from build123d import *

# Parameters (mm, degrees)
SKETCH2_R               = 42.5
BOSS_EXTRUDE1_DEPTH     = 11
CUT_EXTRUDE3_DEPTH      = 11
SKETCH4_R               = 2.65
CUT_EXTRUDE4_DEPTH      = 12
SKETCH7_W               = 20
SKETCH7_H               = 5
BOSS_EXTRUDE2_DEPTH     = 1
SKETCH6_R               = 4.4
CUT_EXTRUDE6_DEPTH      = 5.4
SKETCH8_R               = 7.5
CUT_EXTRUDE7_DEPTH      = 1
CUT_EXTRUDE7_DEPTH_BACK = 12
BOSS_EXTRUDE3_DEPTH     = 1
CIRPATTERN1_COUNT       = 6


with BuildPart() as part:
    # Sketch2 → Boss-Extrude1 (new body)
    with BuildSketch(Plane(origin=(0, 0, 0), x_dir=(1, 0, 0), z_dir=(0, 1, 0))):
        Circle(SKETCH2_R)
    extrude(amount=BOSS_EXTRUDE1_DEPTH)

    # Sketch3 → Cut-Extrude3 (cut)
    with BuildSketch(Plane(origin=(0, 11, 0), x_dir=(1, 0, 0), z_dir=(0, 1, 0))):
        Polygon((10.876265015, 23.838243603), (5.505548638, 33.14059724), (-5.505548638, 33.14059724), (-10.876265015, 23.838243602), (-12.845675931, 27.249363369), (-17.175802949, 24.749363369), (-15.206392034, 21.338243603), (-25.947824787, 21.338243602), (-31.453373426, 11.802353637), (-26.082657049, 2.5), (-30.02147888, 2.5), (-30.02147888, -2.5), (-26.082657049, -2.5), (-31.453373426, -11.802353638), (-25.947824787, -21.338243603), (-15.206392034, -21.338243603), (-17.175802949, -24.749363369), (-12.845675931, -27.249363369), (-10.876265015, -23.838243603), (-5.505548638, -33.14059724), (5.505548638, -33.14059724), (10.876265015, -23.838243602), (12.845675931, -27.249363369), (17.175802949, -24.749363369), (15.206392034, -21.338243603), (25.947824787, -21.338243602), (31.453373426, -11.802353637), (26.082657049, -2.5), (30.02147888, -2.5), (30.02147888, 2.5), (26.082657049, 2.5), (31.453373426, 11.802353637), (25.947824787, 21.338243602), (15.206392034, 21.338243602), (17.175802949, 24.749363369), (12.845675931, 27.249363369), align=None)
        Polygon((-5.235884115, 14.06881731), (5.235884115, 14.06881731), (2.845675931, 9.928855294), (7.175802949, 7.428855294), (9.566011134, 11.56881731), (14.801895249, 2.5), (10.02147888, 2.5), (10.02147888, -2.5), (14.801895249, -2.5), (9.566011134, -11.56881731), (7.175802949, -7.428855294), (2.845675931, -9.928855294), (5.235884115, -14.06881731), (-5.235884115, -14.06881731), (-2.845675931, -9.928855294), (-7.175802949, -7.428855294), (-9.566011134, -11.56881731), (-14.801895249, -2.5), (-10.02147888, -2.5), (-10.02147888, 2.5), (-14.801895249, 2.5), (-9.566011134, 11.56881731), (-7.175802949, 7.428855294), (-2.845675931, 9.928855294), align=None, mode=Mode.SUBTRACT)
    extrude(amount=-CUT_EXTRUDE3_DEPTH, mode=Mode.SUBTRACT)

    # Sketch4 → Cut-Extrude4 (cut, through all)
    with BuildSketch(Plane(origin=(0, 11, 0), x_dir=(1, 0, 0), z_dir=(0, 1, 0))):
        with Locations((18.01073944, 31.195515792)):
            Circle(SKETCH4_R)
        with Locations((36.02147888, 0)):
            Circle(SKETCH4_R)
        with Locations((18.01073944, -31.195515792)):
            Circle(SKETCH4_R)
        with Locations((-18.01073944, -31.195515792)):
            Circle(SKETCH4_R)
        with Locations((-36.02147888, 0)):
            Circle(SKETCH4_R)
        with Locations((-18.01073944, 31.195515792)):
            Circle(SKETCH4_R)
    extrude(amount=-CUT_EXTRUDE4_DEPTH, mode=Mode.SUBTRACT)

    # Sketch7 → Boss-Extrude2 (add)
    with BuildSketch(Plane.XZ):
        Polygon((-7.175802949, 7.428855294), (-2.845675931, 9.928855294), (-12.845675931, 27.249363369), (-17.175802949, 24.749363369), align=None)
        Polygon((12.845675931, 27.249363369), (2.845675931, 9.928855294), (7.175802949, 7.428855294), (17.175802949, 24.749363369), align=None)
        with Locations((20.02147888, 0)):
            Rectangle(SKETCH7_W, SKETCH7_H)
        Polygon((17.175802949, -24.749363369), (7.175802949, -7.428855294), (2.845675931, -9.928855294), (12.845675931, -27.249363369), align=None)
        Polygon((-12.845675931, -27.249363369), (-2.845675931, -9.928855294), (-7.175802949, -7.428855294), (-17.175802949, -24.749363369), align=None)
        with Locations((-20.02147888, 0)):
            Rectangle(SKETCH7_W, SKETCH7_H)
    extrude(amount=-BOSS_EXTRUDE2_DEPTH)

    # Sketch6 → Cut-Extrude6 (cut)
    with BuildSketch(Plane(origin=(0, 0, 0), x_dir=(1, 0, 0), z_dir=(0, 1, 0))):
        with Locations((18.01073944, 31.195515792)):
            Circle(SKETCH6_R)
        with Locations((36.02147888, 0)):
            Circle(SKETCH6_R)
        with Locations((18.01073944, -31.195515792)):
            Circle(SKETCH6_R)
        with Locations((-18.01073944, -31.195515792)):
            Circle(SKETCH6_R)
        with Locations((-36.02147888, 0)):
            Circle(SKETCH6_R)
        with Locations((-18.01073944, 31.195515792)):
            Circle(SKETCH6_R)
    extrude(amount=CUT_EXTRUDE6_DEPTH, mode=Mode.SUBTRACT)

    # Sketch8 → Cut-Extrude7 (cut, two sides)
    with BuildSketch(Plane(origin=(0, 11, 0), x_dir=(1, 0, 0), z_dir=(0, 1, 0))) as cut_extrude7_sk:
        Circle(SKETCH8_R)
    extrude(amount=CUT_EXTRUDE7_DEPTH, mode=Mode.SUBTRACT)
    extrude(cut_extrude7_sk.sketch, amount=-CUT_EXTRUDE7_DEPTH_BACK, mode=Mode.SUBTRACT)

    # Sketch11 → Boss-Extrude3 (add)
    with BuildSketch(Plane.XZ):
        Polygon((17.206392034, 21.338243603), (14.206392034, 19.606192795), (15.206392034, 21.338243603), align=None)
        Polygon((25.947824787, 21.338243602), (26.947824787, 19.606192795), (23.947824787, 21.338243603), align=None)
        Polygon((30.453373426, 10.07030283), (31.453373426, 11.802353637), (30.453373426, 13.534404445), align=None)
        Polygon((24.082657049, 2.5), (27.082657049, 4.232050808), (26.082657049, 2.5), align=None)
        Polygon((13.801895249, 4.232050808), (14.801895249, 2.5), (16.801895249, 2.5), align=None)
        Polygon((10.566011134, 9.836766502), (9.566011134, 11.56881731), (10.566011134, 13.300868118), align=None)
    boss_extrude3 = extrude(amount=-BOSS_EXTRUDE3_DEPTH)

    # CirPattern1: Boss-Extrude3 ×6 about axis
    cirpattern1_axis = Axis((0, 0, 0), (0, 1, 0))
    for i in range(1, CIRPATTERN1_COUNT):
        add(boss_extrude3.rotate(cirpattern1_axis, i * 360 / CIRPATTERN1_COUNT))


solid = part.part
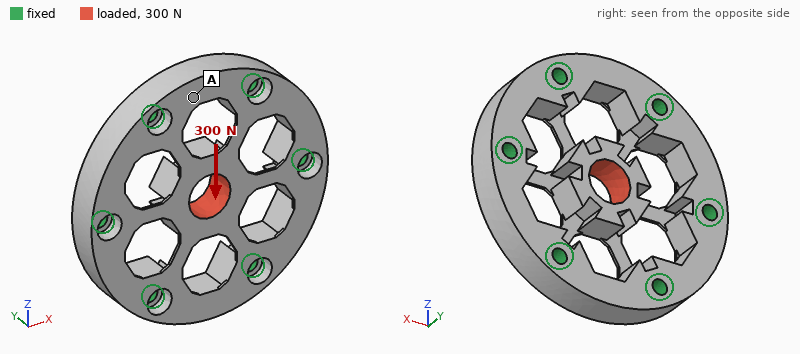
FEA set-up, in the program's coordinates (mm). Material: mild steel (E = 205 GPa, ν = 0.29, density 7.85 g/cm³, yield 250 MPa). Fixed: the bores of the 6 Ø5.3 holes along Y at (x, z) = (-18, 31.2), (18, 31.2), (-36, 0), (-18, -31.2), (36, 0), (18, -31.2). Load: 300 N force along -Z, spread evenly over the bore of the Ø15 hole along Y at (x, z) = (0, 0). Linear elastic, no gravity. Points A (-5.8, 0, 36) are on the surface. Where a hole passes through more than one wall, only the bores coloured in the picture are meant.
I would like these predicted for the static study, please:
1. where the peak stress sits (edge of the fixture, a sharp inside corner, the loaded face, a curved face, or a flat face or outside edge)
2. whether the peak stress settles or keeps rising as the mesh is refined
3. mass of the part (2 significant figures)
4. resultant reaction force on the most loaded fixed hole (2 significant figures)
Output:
a sharp inside corner
keeps rising
250 g
61 N
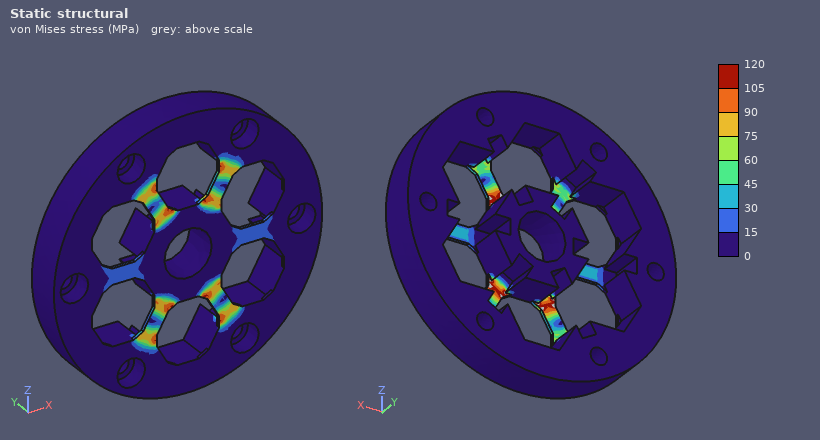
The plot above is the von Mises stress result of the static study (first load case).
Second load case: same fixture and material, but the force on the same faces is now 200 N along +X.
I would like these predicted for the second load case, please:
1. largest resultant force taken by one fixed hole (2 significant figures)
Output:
45 N
